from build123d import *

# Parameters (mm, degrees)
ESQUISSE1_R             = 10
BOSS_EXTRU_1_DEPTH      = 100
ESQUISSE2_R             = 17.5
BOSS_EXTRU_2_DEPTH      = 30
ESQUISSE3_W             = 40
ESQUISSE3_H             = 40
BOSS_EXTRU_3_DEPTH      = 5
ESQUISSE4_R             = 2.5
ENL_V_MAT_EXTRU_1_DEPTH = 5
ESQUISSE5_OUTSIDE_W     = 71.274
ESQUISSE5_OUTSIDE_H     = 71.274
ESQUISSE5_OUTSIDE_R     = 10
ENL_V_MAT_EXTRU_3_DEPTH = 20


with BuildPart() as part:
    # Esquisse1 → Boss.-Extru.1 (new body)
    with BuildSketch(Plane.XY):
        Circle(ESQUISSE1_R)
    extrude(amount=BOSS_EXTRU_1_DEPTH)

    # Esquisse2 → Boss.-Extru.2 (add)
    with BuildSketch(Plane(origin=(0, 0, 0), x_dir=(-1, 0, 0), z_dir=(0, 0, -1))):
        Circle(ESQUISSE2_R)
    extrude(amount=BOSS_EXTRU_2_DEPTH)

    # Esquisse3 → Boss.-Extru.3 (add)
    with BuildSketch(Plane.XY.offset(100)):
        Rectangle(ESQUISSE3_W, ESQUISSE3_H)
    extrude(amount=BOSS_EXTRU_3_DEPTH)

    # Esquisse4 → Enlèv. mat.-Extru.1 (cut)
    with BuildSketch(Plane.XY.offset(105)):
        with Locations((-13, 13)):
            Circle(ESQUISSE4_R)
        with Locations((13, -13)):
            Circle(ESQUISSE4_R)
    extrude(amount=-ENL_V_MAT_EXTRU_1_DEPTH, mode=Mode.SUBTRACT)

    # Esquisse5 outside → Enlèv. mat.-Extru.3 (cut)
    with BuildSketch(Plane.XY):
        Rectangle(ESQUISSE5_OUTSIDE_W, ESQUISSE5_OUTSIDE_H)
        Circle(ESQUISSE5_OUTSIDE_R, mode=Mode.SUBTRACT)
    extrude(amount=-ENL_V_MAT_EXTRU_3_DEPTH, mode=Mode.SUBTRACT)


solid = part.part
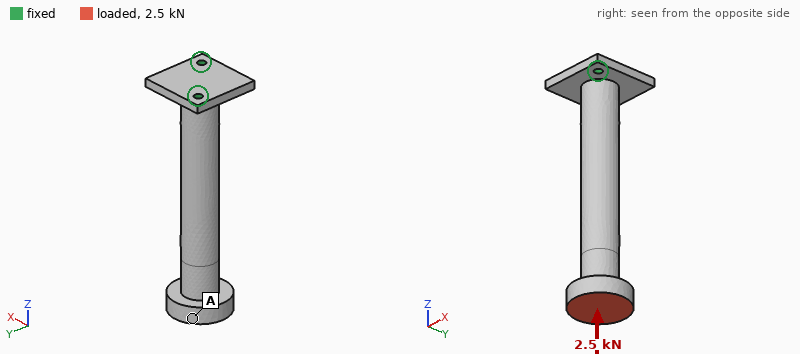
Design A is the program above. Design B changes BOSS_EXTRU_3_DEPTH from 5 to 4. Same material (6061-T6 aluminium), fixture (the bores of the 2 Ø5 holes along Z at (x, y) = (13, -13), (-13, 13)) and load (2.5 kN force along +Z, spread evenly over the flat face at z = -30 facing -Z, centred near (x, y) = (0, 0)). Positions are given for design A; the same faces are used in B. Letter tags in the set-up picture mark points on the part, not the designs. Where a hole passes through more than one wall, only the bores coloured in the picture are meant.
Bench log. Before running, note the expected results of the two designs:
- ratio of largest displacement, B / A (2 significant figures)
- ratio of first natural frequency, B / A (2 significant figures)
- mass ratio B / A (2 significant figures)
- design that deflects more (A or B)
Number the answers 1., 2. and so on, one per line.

1. 1.2
2. 0.81
3. 0.97
4. B
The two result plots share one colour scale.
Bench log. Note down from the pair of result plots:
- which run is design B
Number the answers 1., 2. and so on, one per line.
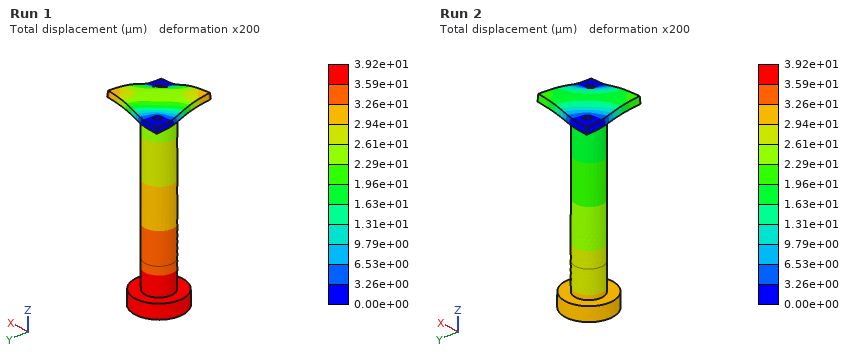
1. Run 1
